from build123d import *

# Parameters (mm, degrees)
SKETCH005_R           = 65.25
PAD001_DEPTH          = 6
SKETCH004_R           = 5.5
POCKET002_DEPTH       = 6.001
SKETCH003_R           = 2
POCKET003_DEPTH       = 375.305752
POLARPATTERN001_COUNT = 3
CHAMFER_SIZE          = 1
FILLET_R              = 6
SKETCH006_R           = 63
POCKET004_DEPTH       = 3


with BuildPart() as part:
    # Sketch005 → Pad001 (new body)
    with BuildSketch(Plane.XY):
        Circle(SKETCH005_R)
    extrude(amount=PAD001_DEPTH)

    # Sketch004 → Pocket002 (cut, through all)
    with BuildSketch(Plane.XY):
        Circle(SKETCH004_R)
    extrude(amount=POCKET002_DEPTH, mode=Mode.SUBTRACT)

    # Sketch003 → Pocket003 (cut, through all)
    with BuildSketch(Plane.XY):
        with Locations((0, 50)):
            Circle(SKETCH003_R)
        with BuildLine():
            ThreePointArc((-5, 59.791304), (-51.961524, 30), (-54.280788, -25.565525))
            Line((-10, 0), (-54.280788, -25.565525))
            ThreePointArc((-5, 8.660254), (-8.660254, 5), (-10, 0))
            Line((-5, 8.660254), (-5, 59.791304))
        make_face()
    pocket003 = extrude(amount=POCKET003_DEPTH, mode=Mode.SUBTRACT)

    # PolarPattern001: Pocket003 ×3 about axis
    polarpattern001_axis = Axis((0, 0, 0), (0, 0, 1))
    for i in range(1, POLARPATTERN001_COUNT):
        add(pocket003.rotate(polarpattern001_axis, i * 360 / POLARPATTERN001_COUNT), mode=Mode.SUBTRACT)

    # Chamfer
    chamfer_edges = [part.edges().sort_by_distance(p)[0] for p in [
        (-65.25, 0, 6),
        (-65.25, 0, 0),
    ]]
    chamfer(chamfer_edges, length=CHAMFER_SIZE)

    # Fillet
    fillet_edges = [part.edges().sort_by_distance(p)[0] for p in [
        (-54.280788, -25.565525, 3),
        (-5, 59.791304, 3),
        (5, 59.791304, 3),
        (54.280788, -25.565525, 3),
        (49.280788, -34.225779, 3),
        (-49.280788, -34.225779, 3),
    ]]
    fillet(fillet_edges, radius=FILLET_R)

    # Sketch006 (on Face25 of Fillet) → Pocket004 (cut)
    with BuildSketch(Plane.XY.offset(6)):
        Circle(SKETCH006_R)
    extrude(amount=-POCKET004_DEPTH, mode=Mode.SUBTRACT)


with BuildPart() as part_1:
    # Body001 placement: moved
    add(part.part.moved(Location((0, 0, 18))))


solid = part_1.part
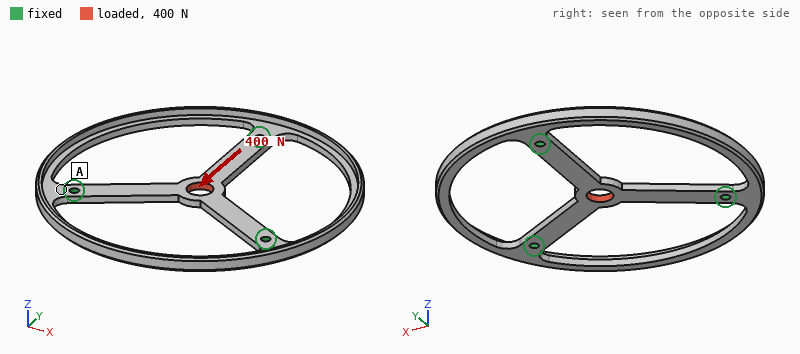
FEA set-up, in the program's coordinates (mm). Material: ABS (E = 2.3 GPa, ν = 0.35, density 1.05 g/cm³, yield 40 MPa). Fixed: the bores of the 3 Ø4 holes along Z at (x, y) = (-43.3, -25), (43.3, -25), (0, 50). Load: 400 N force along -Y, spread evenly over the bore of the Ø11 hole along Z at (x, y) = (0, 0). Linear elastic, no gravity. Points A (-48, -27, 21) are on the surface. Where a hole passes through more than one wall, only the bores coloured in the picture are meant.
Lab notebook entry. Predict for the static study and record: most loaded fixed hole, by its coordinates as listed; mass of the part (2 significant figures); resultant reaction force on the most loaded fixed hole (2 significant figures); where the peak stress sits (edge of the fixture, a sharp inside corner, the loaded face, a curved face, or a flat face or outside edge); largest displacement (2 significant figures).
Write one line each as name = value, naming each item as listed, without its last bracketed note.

most loaded fixed hole, by its coordinates as listed = (0, 50)
mass of the part = 14 g
resultant reaction force on the most loaded fixed hole = 270 N
where the peak stress sits = the loaded face
largest displacement = 0.33 mm
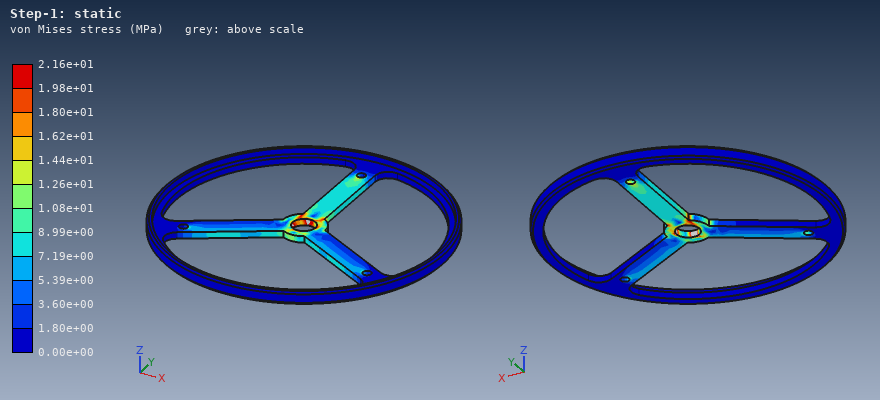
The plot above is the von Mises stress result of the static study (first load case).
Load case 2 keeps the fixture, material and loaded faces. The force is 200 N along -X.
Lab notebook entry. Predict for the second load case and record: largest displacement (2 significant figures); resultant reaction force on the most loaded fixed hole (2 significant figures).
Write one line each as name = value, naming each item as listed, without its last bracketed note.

largest displacement = 0.16 mm
resultant reaction force on the most loaded fixed hole = 120 N
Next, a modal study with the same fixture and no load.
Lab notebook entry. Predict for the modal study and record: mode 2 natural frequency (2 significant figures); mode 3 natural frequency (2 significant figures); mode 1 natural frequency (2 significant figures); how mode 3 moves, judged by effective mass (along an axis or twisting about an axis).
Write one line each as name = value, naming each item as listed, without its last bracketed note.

mode 2 natural frequency = 280 Hz
mode 3 natural frequency = 420 Hz
mode 1 natural frequency = 280 Hz
how mode 3 moves, judged by effective mass = along Z
